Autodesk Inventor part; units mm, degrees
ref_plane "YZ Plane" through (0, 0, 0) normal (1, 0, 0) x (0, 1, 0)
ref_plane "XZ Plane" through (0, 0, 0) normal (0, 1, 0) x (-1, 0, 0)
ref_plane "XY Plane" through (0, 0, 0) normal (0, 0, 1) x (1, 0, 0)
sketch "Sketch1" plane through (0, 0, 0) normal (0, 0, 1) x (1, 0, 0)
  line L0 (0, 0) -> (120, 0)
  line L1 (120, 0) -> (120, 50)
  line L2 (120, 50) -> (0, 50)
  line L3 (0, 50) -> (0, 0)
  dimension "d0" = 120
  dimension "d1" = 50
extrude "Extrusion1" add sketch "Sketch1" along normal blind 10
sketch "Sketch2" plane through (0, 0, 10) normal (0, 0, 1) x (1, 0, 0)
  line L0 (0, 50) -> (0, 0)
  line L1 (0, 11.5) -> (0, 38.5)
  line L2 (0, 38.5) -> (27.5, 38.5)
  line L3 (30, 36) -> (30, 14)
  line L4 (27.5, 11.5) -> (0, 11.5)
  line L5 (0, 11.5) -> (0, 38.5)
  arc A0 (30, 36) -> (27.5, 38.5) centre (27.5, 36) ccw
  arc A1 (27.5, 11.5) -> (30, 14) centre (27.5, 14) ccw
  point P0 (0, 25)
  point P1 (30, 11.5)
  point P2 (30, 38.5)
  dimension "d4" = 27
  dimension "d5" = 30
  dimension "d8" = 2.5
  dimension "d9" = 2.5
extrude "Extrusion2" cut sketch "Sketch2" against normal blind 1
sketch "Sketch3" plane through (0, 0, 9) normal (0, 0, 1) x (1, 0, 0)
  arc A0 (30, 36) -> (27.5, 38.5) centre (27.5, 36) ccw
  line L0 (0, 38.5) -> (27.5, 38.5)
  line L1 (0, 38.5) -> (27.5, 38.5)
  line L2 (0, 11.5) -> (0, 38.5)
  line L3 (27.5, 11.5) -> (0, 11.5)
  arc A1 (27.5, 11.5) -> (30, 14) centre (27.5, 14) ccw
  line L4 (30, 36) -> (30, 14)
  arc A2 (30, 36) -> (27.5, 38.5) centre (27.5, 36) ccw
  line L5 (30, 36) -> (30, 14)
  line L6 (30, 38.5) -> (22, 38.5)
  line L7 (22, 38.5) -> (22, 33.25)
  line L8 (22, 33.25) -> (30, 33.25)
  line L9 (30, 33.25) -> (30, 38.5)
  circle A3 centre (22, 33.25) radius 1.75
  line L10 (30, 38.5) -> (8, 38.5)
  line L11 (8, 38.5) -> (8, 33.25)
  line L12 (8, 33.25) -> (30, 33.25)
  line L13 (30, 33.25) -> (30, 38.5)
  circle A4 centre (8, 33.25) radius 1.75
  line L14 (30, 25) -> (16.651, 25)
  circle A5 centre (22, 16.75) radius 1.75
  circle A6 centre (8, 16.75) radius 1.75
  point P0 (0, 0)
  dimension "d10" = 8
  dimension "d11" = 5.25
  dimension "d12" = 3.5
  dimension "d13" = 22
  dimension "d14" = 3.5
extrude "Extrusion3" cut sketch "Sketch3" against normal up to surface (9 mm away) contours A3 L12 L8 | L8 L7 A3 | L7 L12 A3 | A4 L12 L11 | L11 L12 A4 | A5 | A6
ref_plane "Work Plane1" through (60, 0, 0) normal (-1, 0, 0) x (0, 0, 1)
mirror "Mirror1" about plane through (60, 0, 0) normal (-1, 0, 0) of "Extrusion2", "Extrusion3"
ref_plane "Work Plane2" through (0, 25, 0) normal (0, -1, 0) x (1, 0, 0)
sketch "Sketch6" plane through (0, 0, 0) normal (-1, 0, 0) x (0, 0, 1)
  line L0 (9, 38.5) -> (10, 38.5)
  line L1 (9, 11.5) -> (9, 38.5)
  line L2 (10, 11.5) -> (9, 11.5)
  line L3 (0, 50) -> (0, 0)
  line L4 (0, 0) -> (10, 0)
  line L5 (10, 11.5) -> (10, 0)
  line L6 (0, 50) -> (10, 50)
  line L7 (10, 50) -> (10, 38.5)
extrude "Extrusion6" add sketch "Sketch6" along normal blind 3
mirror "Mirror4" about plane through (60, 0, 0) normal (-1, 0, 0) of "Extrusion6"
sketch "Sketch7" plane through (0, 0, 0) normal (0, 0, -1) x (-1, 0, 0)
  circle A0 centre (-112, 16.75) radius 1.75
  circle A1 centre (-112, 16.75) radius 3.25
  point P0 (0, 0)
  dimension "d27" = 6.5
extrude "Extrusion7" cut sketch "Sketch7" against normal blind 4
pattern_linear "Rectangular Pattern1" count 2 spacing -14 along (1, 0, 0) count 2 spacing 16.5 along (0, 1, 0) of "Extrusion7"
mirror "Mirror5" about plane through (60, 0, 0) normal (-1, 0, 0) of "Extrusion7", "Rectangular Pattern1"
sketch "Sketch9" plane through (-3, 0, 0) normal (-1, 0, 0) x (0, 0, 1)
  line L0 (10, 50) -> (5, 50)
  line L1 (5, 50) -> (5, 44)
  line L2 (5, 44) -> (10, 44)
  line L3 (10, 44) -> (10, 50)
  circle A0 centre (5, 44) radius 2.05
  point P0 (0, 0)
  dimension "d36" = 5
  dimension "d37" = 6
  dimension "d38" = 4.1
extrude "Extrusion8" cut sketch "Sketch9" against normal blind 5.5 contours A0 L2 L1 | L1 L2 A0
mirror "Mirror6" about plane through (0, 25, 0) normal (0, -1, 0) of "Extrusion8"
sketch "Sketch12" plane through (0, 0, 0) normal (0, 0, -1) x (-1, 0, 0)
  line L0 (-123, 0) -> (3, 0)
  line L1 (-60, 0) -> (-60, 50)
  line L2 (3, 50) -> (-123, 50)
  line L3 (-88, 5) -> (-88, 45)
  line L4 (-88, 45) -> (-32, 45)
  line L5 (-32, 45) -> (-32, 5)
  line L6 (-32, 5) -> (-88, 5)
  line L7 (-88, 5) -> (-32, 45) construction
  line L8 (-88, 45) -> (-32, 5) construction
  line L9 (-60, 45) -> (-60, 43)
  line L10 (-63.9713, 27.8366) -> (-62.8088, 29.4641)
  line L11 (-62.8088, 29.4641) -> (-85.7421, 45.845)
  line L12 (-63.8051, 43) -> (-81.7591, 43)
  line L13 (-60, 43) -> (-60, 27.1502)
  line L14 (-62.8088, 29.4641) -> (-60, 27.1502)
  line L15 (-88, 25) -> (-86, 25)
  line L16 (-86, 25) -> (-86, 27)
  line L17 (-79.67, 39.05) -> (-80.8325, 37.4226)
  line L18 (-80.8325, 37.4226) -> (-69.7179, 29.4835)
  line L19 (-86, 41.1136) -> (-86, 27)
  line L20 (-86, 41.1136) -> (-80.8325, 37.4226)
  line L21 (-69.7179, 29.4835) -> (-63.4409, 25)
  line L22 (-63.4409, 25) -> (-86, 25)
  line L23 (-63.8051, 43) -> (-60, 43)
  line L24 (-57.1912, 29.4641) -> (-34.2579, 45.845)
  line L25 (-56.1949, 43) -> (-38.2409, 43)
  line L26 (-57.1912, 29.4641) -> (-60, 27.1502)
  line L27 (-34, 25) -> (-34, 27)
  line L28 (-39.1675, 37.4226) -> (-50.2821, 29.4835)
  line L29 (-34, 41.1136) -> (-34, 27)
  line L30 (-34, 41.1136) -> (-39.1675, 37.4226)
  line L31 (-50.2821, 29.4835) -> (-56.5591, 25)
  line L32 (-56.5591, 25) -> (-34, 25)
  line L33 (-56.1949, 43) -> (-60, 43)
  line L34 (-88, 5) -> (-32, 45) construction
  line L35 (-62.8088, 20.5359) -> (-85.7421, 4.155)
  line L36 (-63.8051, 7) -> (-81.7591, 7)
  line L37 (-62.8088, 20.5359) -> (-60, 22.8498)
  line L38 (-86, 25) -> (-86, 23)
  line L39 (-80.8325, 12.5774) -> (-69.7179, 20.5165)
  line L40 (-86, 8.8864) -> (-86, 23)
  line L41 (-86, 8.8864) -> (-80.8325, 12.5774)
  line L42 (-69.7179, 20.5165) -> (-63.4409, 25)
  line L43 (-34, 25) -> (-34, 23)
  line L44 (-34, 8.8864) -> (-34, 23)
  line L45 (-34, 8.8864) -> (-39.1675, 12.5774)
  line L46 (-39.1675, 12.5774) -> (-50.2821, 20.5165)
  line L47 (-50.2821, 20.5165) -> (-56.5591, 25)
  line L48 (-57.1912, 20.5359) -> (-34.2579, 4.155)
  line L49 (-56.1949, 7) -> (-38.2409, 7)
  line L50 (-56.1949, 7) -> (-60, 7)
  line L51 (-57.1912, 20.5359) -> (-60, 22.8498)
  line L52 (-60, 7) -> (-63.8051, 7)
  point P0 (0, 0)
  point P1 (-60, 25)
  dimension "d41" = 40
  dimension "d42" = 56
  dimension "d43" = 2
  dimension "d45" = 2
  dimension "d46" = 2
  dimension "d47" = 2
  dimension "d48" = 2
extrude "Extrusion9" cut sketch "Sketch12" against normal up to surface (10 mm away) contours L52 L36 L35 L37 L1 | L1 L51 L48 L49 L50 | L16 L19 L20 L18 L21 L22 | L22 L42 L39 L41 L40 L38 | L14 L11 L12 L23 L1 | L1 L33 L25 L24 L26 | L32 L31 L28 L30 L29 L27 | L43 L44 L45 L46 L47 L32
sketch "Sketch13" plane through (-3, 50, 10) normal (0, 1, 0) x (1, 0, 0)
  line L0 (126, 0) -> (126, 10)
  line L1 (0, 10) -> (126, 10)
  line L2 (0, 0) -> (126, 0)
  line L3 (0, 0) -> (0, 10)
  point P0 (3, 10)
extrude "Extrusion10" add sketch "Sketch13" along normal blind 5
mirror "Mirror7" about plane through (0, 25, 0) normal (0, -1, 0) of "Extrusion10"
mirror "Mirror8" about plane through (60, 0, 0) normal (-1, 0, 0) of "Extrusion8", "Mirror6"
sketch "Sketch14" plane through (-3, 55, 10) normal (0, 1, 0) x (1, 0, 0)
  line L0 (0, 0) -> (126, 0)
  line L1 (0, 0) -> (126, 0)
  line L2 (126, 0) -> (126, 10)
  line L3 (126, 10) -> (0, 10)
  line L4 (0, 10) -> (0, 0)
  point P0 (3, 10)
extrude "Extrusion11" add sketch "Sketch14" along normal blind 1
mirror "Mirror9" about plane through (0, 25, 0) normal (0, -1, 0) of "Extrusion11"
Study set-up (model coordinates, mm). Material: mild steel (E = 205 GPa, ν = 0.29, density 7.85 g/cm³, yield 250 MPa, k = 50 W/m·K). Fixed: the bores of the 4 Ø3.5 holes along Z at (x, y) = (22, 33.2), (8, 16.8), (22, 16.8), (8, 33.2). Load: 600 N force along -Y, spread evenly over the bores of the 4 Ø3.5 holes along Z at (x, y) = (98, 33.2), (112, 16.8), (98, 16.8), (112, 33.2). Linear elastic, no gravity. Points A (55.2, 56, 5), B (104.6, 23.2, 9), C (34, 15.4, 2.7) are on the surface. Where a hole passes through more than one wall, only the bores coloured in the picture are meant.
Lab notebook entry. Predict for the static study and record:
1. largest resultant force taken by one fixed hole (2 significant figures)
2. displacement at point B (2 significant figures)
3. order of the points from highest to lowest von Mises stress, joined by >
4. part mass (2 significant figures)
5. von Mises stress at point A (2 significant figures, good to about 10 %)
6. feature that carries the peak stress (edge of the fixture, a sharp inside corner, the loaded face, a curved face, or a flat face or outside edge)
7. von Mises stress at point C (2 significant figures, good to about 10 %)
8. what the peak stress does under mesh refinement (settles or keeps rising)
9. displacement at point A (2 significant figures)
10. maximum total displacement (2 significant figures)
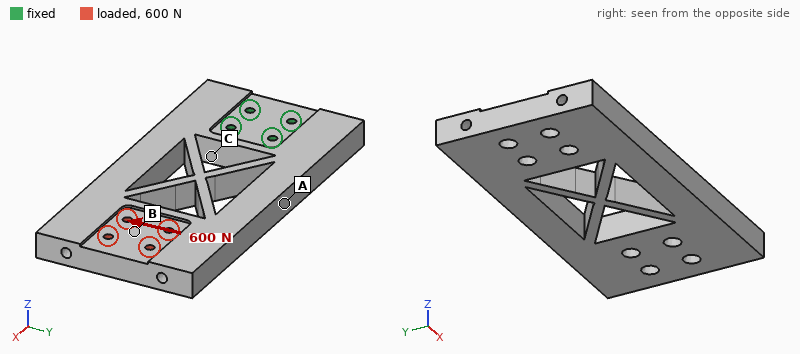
1.3 kN
15 µm
C > A > B
480 g
6.2 MPa
edge of the fixture
9.9 MPa
keeps rising
7.0 µm
18 µm
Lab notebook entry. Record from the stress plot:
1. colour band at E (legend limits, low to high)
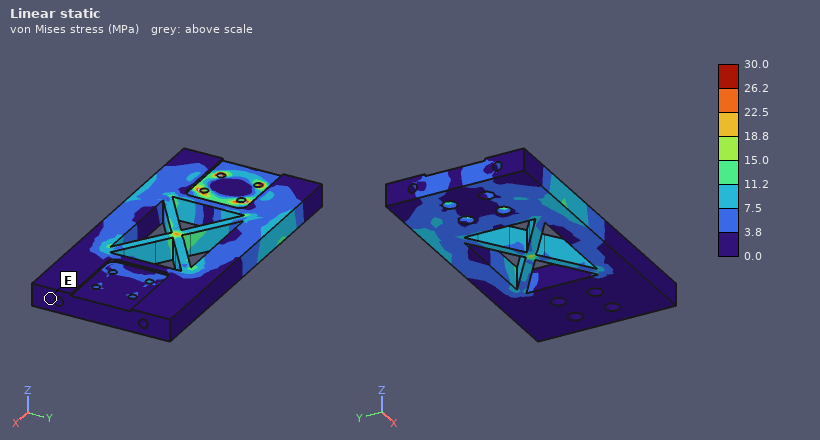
0.0 to 3.8 MPa
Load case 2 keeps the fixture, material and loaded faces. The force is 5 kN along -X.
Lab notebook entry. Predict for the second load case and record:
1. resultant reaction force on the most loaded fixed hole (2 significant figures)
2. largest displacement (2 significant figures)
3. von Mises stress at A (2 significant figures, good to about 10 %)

1.5 kN
73 µm
9.1 MPa
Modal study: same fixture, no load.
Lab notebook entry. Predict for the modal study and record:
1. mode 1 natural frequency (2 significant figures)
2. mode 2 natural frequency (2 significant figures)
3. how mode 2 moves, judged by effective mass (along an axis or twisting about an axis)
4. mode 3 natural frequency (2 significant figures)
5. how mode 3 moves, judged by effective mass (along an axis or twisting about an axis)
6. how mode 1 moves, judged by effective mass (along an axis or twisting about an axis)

570 Hz
1800 Hz
twisting about X
2200 Hz
along Y
along Z
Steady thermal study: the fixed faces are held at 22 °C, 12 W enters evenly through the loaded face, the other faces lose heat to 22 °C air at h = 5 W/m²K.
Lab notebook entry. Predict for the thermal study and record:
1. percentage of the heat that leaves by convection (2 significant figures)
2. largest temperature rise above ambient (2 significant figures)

23 %
55 K
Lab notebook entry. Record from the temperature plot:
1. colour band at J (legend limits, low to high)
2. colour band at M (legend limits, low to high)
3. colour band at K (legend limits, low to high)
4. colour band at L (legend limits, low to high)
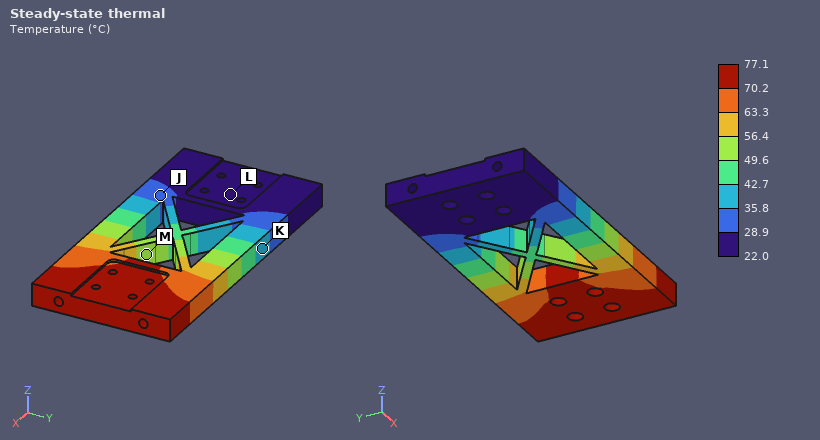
28.9 to 35.8 °C
49.6 to 56.4 °C
35.8 to 42.7 °C
22.0 to 28.9 °C
